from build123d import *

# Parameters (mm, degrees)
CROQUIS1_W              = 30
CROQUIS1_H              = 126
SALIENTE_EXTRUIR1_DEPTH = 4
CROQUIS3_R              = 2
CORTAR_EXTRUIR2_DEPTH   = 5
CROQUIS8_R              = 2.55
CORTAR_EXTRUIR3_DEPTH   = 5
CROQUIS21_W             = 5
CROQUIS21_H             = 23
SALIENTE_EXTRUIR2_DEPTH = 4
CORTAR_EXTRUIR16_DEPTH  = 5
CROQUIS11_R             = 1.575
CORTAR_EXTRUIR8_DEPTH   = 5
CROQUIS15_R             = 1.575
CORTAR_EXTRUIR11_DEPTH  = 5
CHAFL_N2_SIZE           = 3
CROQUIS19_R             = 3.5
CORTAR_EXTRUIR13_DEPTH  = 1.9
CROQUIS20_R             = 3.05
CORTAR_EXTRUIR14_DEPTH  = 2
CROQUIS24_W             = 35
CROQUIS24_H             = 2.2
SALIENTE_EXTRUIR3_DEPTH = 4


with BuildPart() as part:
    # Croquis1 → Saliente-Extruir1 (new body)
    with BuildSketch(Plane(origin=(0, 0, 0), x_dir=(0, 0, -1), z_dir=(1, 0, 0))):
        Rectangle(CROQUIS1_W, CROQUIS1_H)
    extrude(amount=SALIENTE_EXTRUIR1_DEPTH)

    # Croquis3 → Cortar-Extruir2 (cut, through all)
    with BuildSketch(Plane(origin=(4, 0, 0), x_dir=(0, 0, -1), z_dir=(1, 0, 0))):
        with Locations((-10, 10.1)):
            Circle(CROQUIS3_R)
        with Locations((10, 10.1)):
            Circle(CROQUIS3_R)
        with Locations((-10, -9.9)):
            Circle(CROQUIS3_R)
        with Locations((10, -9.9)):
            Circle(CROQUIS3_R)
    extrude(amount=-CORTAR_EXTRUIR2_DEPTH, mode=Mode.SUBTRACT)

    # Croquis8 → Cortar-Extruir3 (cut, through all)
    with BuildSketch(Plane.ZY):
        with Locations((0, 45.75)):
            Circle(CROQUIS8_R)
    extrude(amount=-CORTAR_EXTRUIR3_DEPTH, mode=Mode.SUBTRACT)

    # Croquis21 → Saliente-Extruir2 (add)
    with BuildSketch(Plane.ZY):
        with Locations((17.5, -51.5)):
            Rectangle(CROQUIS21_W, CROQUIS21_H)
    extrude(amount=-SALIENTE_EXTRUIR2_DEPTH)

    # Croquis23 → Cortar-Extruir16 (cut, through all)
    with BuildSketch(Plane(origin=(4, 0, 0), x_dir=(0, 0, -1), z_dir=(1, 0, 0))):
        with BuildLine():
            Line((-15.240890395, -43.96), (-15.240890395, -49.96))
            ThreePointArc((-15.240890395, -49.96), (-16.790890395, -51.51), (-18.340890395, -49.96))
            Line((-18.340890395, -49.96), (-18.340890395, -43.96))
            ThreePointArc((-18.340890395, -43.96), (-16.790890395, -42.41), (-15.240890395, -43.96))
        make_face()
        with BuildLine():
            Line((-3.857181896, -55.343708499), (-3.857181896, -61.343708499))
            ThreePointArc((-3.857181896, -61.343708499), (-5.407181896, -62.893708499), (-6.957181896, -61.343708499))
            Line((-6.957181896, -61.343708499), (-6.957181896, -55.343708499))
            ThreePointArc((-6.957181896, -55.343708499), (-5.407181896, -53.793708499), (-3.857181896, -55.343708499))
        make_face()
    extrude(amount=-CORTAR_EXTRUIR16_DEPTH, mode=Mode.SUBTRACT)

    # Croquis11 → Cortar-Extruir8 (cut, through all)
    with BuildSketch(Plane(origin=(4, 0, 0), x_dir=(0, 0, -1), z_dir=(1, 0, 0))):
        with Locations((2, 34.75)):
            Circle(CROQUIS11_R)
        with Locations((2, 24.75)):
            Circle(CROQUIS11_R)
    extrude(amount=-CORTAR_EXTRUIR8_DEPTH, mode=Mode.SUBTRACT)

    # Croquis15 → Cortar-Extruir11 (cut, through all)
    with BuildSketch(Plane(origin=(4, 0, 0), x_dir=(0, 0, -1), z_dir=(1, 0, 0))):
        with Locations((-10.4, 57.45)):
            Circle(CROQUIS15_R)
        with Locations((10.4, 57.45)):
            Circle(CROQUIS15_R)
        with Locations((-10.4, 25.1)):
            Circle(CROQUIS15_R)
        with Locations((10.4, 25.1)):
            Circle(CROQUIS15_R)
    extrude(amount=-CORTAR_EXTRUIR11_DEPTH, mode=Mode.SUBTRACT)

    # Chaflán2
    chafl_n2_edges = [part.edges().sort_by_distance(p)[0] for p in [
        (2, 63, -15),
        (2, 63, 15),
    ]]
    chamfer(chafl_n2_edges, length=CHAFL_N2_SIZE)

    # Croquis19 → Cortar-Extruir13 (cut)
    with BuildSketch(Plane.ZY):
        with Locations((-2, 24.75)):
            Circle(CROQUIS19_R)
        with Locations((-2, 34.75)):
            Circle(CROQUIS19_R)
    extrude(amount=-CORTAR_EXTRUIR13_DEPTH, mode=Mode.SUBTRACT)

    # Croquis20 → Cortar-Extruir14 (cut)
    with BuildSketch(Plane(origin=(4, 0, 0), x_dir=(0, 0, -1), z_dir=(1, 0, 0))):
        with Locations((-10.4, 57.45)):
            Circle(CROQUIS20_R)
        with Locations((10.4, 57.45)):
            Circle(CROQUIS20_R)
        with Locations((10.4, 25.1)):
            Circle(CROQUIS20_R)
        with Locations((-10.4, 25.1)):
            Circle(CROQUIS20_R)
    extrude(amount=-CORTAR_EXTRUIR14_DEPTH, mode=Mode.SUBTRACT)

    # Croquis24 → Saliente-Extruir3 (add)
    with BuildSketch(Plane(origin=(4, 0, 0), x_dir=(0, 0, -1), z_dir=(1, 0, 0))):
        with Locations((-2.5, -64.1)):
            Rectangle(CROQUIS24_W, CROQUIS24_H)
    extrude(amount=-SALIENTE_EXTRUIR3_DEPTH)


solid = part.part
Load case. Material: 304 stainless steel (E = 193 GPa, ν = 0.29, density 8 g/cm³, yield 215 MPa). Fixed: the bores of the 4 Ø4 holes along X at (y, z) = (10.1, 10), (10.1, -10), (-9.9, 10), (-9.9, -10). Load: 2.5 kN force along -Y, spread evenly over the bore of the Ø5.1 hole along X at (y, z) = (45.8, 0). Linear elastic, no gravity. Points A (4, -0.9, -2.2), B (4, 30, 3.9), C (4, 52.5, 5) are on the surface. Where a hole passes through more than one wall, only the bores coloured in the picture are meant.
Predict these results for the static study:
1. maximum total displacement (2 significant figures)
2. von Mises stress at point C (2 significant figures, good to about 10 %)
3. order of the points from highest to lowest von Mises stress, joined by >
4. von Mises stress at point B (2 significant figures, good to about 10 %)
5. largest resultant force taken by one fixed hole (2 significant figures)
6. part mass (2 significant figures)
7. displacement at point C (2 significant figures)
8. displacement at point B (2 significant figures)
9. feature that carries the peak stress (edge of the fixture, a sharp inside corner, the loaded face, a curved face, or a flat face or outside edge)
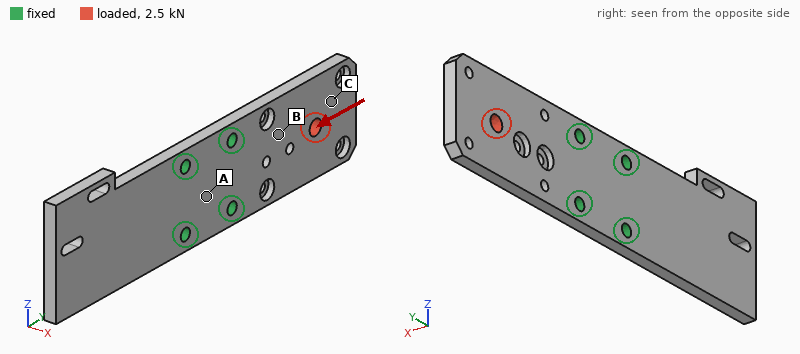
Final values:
6.5 µm
15 MPa
B > C > A
37 MPa
1.1 kN
120 g
5.4 µm
3.1 µm
a curved face
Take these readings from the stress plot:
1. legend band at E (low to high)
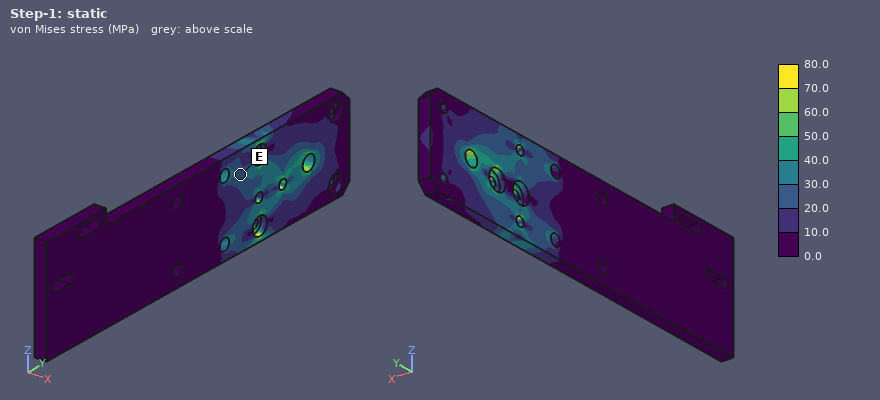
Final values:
20.0 to 30.0 MPa
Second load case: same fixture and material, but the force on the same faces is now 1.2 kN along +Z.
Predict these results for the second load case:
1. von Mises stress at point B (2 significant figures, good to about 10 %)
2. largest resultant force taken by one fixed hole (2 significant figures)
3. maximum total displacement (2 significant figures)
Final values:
20 MPa
1.9 kN
31 µm
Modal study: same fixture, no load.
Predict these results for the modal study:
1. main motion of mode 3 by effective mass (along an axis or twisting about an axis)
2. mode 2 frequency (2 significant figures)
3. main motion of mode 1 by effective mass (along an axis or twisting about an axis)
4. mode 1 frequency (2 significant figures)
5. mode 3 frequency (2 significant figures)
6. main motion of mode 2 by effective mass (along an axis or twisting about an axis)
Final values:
twisting about Y
1100 Hz
along X
1000 Hz
3400 Hz
along X
